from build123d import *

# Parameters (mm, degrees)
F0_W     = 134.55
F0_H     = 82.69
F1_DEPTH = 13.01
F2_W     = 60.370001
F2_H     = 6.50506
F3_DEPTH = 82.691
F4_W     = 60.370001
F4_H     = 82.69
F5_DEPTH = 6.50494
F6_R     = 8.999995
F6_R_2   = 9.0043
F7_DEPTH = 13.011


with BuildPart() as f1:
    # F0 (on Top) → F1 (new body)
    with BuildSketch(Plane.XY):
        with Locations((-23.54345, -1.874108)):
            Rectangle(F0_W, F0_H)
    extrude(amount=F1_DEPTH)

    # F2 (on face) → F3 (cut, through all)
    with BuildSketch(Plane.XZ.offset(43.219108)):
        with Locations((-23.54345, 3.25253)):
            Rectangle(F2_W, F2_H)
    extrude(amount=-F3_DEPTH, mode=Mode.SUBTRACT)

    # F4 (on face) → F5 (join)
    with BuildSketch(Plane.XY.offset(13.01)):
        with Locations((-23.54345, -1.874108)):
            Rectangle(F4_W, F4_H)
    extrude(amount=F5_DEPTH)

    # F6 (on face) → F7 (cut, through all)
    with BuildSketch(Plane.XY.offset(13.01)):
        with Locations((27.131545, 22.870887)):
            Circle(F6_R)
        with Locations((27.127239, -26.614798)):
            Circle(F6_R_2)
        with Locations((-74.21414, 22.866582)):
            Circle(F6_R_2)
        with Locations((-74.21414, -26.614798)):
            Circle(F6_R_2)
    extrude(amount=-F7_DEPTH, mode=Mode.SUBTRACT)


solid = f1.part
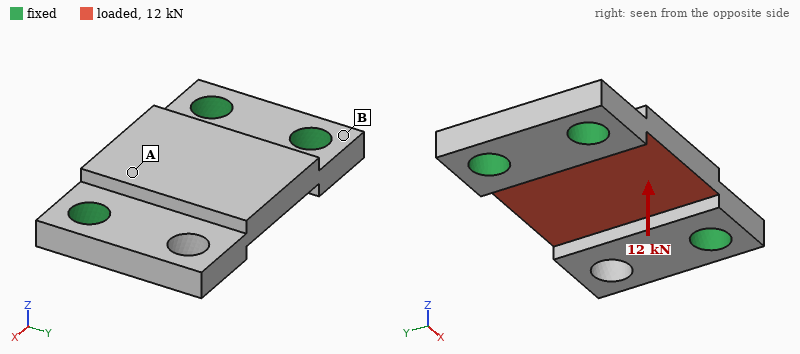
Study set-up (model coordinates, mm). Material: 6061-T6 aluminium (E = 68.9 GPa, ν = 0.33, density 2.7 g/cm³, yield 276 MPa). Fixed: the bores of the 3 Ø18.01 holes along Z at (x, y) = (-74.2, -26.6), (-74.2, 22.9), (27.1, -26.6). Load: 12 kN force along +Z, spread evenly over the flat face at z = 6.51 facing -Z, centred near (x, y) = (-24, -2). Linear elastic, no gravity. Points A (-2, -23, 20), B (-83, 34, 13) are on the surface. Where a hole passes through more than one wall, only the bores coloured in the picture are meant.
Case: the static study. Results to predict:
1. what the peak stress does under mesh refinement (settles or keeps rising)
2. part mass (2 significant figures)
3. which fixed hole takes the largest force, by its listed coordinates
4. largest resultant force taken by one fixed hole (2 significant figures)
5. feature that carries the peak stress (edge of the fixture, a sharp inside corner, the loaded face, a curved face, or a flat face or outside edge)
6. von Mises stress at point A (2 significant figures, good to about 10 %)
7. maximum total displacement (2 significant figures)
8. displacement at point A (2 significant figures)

keeps rising
360 g
(27.1, -26.6)
8.5 kN
edge of the fixture
25 MPa
0.12 mm
0.028 mm
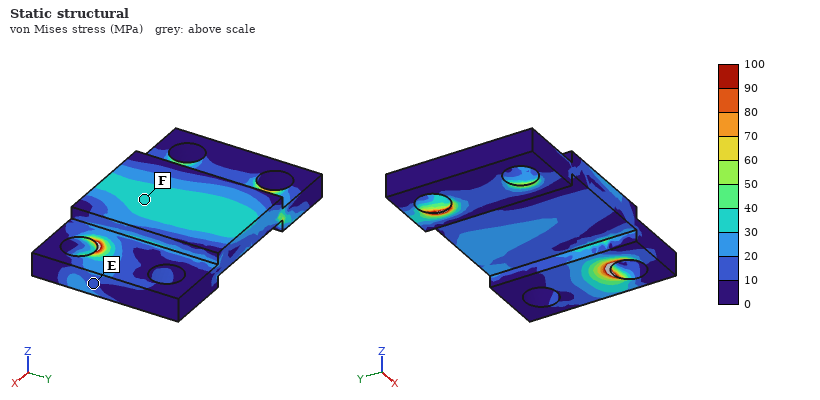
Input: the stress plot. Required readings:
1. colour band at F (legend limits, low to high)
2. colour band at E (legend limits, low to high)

30 to 40 MPa
10 to 20 MPa
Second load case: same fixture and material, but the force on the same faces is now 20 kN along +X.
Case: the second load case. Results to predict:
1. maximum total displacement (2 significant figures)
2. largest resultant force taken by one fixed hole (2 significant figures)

34 µm
7.0 kN
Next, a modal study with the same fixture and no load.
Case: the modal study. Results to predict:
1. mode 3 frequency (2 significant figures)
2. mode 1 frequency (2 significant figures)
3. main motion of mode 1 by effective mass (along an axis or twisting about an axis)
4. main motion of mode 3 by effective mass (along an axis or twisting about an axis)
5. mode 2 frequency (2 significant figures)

8500 Hz
3500 Hz
along Z
along Z
6300 Hz
